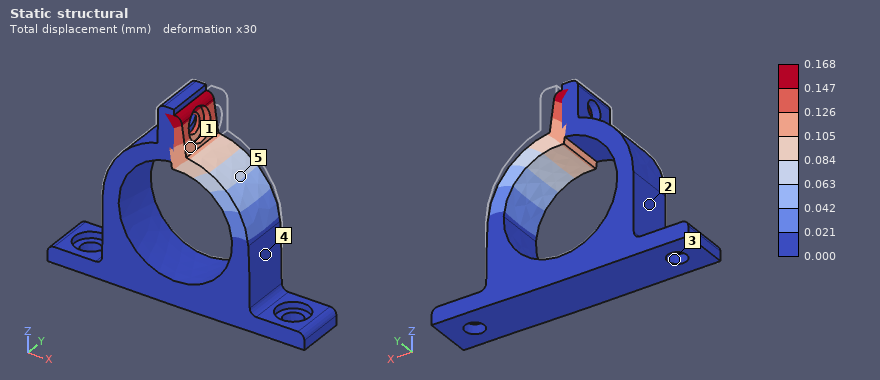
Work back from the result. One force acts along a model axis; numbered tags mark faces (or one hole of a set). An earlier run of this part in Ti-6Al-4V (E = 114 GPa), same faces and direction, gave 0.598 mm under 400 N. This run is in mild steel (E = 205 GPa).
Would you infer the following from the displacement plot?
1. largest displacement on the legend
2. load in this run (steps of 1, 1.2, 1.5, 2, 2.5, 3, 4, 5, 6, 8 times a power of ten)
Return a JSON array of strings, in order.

["0.168 mm", "200 N"]
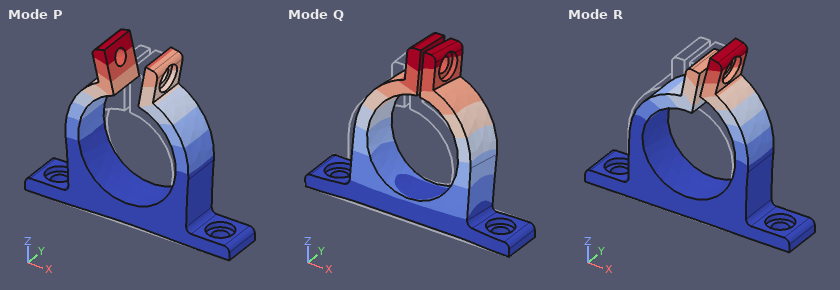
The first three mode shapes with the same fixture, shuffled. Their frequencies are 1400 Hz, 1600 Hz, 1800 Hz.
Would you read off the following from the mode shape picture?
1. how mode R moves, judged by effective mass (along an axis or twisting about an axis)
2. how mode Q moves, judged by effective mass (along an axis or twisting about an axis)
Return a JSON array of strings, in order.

["along X", "along Y"]
